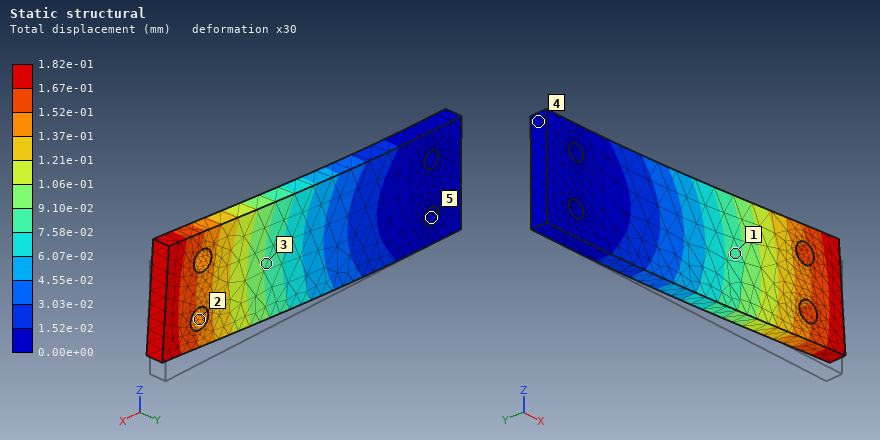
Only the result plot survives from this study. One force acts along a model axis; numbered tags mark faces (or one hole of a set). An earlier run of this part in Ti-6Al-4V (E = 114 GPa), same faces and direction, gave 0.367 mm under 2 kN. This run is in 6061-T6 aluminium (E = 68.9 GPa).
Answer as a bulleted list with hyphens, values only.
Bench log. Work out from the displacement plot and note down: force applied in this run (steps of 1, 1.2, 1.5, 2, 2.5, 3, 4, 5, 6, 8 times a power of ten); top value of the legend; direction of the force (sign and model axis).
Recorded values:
- 600 N
- 1.82e-01 mm
- +Z
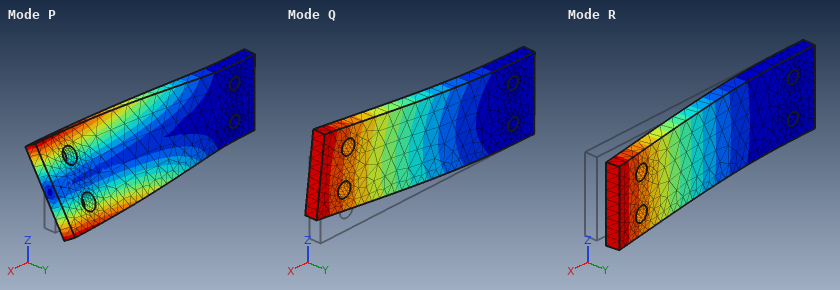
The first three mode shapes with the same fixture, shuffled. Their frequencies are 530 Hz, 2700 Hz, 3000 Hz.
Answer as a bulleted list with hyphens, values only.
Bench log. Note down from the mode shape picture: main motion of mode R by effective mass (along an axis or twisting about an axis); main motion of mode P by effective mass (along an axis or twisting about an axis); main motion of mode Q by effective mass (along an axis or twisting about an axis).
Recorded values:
- along Y
- twisting about X
- along Z
